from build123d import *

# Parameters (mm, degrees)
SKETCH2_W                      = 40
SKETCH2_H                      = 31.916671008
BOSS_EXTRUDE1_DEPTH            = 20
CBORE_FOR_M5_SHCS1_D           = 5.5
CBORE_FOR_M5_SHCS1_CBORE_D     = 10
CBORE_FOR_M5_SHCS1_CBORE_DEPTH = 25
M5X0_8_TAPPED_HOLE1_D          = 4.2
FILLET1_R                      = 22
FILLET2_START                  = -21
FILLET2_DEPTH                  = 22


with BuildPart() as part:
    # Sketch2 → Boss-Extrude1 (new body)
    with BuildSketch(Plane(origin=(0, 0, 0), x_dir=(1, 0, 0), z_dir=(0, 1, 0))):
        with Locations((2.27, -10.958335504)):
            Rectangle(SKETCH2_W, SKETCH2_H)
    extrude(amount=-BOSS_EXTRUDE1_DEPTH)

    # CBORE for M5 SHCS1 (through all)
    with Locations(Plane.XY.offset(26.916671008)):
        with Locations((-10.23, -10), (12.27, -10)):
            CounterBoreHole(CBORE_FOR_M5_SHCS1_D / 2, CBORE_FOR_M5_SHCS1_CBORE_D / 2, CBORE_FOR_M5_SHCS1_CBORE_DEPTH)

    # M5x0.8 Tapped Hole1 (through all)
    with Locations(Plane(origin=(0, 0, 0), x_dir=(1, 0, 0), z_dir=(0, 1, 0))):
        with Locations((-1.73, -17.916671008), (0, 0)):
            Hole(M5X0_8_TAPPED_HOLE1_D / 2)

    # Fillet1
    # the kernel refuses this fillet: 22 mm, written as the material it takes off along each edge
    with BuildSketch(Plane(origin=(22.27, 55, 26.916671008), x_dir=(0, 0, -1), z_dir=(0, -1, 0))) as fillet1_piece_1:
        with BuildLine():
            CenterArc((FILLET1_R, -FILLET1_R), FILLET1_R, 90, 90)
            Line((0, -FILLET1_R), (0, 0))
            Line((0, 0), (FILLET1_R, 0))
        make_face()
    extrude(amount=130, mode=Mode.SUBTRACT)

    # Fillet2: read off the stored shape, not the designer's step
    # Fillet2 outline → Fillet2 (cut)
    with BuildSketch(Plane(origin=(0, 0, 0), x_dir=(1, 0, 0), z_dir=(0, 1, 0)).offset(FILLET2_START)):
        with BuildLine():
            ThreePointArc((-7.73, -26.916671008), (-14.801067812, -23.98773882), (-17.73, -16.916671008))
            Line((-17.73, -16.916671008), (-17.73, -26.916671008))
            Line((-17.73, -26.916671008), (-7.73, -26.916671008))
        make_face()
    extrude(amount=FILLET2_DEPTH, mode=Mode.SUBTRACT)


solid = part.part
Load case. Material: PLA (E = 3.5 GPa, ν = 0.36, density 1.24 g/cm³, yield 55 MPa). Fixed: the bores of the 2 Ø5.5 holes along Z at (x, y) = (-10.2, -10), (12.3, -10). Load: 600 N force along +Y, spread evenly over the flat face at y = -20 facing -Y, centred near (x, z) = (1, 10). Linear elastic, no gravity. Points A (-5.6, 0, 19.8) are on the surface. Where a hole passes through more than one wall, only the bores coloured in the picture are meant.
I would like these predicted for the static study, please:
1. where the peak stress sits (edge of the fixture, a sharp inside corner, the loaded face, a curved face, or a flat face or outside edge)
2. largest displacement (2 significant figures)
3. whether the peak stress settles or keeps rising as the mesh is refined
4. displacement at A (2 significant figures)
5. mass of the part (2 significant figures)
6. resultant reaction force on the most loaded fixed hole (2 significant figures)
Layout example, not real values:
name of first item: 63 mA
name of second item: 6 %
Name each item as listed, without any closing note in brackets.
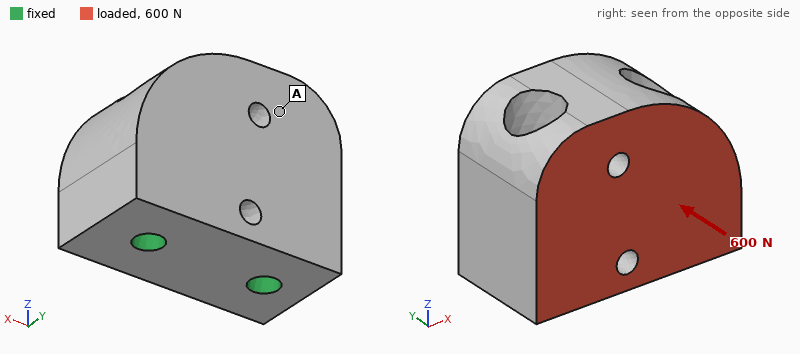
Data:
where the peak stress sits: edge of the fixture
largest displacement: 0.15 mm
whether the peak stress settles or keeps rising as the mesh is refined: keeps rising
displacement at A: 0.11 mm
mass of the part: 23 g
resultant reaction force on the most loaded fixed hole: 310 N
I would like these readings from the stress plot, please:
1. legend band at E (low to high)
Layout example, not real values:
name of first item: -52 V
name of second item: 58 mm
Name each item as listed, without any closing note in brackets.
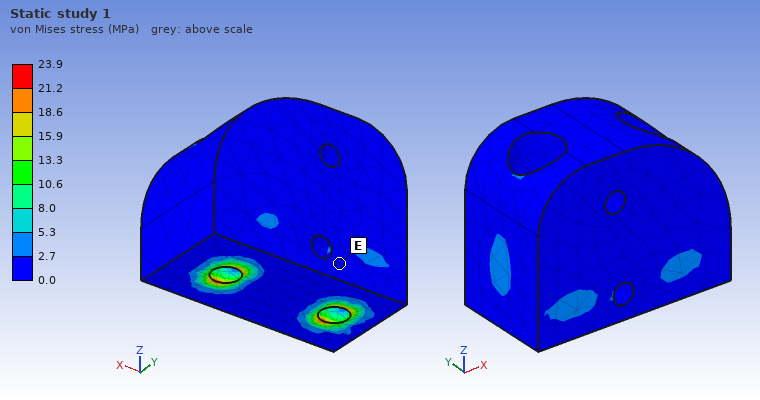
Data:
legend band at E: 0.0 to 2.7 MPa
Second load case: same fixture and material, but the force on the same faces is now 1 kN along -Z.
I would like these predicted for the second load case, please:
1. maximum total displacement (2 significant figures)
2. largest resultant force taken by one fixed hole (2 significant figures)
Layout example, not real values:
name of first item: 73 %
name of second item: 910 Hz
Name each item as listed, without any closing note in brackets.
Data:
maximum total displacement: 0.21 mm
largest resultant force taken by one fixed hole: 510 N
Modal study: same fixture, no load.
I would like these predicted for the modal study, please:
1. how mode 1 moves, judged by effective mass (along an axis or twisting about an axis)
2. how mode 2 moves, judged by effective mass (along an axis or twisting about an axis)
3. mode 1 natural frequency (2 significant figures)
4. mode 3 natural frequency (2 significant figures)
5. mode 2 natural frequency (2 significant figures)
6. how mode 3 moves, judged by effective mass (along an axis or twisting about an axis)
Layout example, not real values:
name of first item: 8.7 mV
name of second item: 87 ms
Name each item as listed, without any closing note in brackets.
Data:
how mode 1 moves, judged by effective mass: along Y
how mode 2 moves, judged by effective mass: along X
mode 1 natural frequency: 2700 Hz
mode 3 natural frequency: 7000 Hz
mode 2 natural frequency: 5200 Hz
how mode 3 moves, judged by effective mass: twisting about Z
